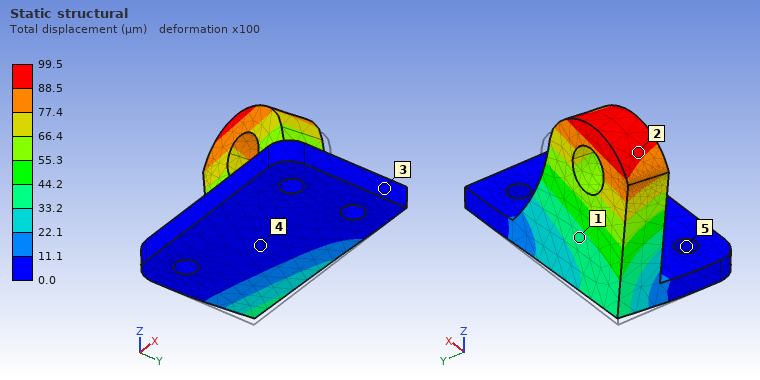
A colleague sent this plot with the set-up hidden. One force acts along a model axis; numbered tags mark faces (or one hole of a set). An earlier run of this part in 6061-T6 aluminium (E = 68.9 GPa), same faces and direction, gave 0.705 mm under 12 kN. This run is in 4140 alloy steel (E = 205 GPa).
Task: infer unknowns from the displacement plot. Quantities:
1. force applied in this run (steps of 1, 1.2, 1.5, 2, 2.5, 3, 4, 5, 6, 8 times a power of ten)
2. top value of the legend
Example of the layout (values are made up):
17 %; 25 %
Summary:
5 kN; 99.5 µm
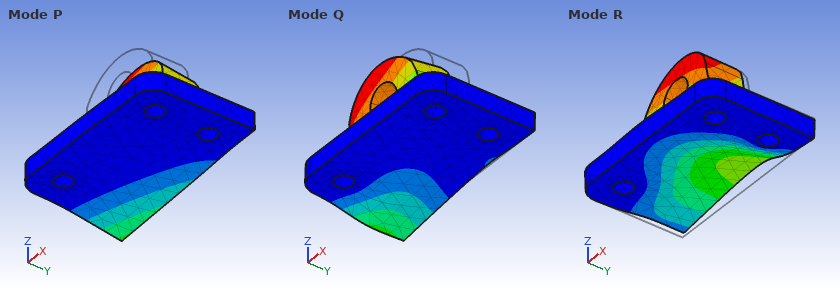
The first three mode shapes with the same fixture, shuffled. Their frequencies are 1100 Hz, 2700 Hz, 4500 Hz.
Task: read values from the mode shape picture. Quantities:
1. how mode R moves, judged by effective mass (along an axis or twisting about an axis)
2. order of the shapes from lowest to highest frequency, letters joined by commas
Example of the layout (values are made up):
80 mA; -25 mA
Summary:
along Z; P, Q, R
